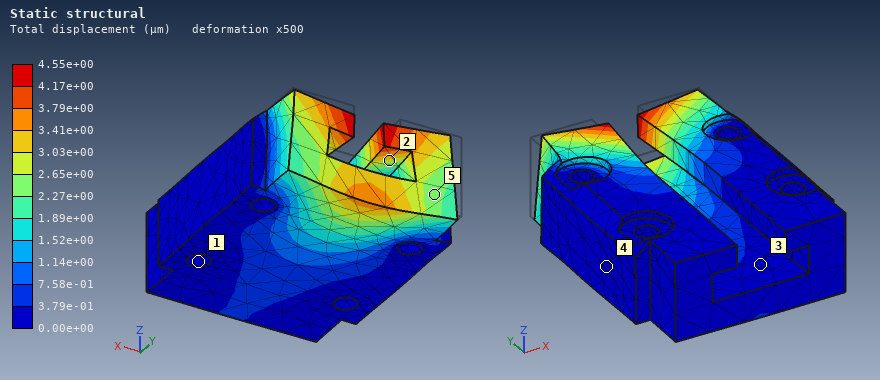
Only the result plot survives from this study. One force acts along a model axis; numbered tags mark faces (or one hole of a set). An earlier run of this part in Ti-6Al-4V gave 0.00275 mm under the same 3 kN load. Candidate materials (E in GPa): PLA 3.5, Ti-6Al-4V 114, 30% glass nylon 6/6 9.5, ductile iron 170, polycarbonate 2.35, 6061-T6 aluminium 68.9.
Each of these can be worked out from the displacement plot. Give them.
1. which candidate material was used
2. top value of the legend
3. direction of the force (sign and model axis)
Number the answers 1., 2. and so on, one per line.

1. 6061-T6 aluminium
2. 4.55e+00 µm
3. -Y
